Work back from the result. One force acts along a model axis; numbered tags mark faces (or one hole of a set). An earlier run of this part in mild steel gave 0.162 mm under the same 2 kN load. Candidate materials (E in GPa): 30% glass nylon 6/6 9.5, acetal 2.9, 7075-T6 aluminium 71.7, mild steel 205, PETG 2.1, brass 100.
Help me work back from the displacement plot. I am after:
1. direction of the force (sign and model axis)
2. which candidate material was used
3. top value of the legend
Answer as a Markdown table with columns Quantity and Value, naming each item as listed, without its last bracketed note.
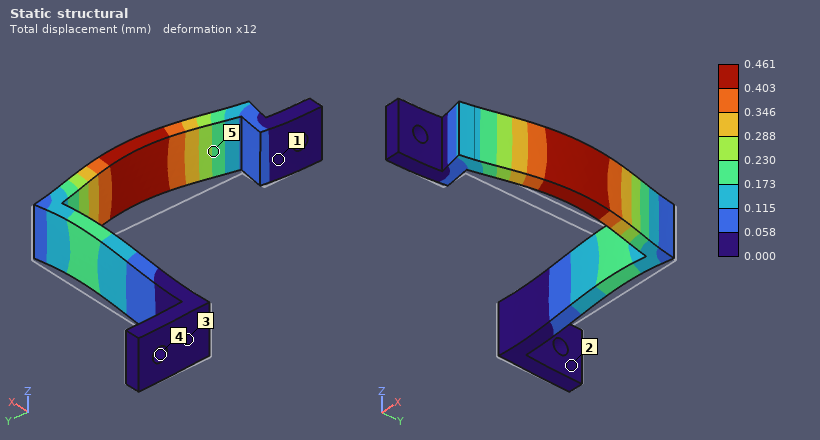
| Quantity | Value |
|---|---|
| direction of the force | +X |
| which candidate material was used | 7075-T6 aluminium |
| top value of the legend | 0.461 mm |
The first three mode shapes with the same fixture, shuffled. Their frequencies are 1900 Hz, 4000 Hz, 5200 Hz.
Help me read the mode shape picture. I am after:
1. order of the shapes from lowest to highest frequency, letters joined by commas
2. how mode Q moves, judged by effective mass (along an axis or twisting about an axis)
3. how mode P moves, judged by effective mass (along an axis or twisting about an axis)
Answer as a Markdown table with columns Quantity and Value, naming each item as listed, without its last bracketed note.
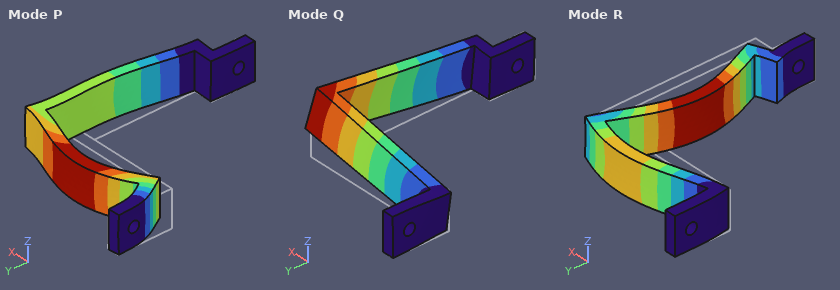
| Quantity | Value |
|---|---|
| order of the shapes from lowest to highest frequency, letters joined by commas | Q, R, P |
| how mode Q moves, judged by effective mass | along Z |
| how mode P moves, judged by effective mass | along X |
